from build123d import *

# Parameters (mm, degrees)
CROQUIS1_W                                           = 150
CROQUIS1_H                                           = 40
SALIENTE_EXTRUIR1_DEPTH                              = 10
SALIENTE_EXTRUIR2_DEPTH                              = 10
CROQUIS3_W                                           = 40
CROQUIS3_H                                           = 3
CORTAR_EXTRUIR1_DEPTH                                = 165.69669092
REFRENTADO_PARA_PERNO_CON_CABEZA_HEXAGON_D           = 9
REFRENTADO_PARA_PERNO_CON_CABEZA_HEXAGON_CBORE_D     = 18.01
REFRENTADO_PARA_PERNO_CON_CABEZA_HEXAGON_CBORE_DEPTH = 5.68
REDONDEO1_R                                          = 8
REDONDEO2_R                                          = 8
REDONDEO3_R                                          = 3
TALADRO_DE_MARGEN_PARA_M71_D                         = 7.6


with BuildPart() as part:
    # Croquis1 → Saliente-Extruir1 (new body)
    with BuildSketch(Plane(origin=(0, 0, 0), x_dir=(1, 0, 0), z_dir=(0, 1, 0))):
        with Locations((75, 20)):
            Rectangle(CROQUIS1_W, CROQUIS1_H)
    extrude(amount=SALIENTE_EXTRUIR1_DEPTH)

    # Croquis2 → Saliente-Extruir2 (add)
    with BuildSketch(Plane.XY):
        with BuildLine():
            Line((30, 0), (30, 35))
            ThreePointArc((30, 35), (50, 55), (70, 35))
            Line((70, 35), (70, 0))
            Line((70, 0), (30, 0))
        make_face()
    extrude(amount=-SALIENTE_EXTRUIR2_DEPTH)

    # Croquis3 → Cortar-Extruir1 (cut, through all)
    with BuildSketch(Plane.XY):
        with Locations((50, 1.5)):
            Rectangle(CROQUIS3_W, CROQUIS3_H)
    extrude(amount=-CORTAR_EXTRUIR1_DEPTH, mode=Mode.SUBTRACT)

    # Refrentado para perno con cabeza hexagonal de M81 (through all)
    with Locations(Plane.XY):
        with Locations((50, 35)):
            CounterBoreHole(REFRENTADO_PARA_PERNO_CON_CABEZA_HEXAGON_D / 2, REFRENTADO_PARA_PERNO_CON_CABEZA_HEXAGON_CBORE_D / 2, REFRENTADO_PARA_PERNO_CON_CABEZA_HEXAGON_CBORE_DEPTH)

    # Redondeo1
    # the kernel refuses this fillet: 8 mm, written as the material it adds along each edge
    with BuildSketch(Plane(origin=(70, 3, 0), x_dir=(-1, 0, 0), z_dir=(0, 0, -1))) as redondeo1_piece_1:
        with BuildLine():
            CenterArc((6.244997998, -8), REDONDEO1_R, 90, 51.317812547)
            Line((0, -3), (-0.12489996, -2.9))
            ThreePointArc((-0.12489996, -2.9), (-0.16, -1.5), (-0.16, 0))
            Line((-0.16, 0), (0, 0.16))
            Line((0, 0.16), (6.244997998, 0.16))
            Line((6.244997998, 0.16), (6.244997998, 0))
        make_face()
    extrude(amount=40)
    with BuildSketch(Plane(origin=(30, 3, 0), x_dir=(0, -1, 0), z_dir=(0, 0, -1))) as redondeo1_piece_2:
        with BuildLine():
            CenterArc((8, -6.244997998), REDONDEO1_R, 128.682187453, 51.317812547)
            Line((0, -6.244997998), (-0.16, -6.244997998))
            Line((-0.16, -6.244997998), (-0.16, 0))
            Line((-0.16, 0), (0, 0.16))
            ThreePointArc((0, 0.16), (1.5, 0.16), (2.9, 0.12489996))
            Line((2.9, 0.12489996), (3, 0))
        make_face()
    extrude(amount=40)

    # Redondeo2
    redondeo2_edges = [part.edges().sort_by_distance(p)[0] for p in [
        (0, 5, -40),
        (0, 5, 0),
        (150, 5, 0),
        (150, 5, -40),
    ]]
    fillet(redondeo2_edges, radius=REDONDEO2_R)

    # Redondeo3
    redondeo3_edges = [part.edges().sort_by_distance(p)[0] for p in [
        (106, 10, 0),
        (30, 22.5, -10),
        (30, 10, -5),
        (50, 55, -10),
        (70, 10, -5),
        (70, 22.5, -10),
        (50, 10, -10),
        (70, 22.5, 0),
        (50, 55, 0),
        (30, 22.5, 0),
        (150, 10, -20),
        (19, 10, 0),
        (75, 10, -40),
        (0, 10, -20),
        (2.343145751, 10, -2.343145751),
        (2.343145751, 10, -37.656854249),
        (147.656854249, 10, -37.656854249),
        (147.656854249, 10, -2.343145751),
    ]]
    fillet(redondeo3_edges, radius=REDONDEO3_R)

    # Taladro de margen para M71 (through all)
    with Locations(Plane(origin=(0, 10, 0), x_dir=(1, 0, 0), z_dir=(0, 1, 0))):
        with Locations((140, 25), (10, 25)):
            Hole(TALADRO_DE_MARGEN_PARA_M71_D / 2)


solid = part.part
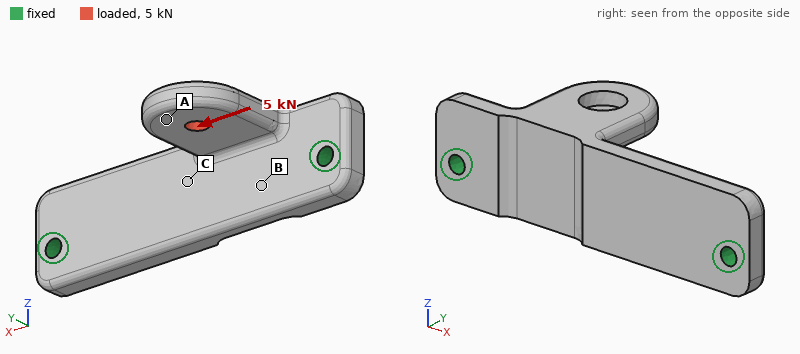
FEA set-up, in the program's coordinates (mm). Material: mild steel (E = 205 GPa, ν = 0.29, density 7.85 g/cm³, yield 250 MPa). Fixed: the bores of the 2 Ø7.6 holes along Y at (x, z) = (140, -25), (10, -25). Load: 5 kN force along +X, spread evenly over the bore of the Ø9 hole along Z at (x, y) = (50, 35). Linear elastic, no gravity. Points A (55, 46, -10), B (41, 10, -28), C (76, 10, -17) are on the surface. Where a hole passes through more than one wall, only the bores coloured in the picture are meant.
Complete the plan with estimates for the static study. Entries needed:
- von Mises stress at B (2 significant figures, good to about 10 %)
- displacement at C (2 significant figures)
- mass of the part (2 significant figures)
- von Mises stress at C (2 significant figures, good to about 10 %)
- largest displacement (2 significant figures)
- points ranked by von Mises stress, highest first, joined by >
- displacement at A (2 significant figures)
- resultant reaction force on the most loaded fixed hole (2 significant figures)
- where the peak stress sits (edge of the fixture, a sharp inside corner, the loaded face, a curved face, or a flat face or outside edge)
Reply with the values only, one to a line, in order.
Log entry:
43 MPa
0.061 mm
530 g
75 MPa
0.13 mm
C > B > A
0.11 mm
3.0 kN
a curved face
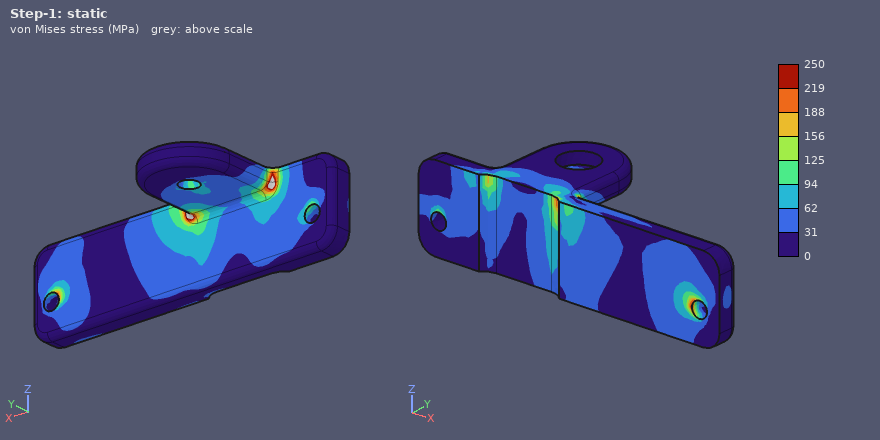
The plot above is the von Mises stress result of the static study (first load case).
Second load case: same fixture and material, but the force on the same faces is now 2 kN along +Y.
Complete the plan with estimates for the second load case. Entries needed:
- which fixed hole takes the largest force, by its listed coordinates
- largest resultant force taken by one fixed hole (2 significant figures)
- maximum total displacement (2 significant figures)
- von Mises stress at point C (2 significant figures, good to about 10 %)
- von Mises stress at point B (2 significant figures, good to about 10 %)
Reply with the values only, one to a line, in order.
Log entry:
(10, -25)
1.6 kN
51 µm
23 MPa
10.0 MPa
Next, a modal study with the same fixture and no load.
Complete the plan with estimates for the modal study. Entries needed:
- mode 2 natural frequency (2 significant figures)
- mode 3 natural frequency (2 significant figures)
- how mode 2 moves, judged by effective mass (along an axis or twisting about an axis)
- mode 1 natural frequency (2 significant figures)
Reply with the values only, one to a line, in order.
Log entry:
2500 Hz
5100 Hz
along Y
2000 Hz
